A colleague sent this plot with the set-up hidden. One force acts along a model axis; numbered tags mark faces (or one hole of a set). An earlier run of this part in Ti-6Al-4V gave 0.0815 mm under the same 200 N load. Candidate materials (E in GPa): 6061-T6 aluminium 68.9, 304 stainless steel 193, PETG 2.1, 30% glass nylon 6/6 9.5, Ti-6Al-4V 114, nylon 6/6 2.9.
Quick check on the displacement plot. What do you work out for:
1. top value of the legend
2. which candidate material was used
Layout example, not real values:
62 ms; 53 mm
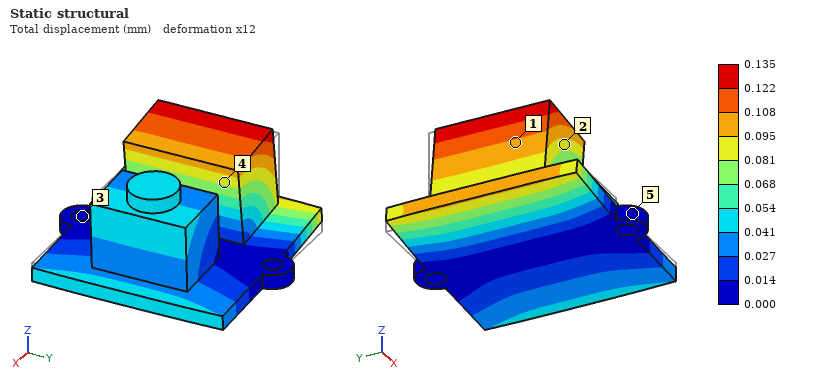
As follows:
0.135 mm; 6061-T6 aluminium
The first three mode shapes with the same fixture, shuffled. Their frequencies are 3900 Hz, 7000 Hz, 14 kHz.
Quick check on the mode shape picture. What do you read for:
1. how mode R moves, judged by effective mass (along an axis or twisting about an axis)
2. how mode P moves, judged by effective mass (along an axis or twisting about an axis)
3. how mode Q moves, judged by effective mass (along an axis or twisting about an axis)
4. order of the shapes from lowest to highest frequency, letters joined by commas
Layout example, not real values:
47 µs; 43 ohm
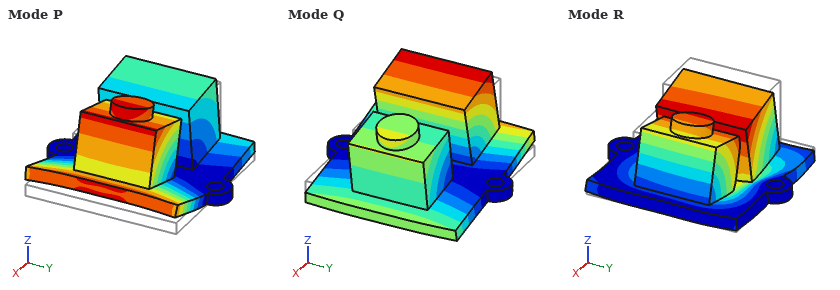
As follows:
along Z; along Z; along X; Q, P, R
